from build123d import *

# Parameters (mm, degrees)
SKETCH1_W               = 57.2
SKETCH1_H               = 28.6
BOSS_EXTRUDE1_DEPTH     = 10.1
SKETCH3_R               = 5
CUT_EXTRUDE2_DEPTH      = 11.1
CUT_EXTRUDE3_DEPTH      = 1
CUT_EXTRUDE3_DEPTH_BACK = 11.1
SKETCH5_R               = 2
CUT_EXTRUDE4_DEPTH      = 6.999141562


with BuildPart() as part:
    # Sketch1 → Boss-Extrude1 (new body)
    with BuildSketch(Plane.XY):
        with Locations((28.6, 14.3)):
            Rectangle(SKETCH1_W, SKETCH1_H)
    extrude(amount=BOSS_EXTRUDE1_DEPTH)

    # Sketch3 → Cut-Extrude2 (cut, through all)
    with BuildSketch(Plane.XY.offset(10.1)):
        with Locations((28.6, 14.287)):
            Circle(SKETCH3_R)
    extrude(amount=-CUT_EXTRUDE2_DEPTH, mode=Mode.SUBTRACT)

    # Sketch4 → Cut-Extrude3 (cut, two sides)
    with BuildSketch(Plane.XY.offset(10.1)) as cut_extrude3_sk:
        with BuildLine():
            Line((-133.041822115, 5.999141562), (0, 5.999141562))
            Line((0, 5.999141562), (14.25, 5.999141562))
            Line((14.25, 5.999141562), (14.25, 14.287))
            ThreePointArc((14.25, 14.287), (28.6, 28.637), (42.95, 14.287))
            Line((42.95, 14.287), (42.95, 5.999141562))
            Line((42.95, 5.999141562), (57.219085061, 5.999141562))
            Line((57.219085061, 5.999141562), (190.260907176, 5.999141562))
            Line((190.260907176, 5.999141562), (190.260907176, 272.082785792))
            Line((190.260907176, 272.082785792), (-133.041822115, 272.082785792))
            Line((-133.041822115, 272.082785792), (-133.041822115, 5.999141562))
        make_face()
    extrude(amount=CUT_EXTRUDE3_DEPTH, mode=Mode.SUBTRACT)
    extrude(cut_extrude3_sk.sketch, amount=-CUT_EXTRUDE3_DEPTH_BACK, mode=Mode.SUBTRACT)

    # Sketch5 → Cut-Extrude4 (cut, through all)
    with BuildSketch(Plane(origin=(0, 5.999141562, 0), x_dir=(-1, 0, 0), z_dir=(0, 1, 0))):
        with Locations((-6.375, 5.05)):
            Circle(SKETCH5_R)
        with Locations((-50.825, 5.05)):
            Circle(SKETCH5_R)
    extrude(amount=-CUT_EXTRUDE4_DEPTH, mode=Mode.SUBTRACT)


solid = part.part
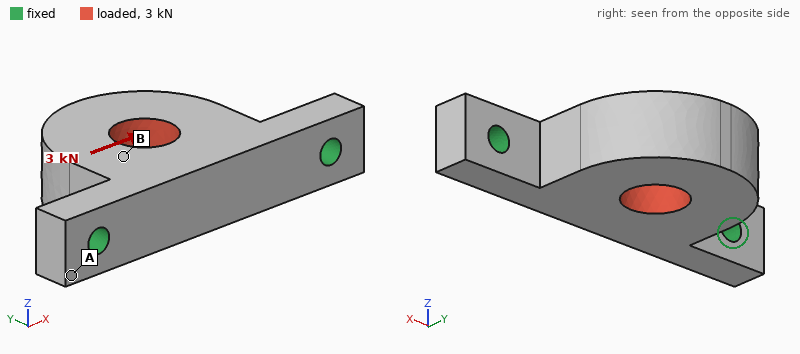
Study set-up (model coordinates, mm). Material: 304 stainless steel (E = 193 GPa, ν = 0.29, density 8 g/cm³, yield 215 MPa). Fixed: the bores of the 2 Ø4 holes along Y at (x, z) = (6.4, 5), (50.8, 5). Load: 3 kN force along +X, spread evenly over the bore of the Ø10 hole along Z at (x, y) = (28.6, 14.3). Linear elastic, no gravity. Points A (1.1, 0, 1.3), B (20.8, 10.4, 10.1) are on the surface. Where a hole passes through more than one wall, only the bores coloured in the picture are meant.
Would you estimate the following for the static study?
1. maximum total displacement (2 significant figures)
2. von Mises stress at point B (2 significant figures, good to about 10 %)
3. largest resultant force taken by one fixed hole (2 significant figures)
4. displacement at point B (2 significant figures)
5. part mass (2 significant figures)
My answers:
9.5 µm
21 MPa
1.8 kN
3.9 µm
66 g
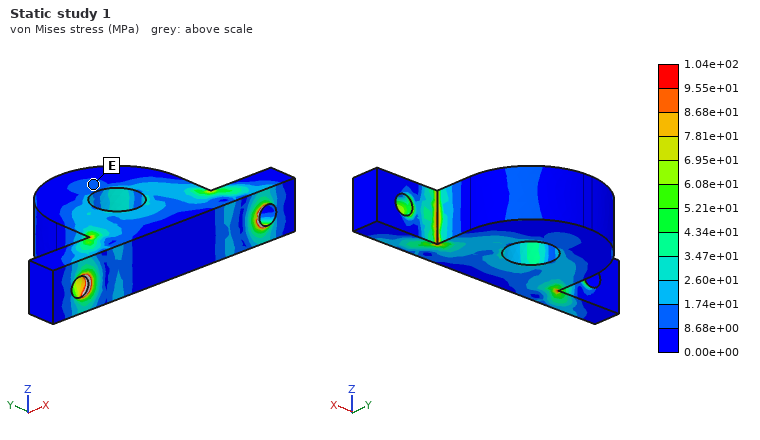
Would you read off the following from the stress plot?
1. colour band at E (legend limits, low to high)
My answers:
8.68e+00 to 1.74e+01 MPa
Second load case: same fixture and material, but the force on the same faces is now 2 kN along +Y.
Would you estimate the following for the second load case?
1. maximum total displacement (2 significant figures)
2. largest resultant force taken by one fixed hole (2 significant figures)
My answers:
6.4 µm
1.1 kN
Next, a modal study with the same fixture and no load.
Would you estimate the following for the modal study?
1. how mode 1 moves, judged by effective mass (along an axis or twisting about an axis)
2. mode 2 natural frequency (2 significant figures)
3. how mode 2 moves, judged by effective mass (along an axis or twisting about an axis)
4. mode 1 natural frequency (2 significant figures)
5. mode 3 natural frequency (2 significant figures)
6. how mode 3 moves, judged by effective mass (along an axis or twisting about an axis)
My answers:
along Z
13 kHz
along Y
4400 Hz
14 kHz
along X
